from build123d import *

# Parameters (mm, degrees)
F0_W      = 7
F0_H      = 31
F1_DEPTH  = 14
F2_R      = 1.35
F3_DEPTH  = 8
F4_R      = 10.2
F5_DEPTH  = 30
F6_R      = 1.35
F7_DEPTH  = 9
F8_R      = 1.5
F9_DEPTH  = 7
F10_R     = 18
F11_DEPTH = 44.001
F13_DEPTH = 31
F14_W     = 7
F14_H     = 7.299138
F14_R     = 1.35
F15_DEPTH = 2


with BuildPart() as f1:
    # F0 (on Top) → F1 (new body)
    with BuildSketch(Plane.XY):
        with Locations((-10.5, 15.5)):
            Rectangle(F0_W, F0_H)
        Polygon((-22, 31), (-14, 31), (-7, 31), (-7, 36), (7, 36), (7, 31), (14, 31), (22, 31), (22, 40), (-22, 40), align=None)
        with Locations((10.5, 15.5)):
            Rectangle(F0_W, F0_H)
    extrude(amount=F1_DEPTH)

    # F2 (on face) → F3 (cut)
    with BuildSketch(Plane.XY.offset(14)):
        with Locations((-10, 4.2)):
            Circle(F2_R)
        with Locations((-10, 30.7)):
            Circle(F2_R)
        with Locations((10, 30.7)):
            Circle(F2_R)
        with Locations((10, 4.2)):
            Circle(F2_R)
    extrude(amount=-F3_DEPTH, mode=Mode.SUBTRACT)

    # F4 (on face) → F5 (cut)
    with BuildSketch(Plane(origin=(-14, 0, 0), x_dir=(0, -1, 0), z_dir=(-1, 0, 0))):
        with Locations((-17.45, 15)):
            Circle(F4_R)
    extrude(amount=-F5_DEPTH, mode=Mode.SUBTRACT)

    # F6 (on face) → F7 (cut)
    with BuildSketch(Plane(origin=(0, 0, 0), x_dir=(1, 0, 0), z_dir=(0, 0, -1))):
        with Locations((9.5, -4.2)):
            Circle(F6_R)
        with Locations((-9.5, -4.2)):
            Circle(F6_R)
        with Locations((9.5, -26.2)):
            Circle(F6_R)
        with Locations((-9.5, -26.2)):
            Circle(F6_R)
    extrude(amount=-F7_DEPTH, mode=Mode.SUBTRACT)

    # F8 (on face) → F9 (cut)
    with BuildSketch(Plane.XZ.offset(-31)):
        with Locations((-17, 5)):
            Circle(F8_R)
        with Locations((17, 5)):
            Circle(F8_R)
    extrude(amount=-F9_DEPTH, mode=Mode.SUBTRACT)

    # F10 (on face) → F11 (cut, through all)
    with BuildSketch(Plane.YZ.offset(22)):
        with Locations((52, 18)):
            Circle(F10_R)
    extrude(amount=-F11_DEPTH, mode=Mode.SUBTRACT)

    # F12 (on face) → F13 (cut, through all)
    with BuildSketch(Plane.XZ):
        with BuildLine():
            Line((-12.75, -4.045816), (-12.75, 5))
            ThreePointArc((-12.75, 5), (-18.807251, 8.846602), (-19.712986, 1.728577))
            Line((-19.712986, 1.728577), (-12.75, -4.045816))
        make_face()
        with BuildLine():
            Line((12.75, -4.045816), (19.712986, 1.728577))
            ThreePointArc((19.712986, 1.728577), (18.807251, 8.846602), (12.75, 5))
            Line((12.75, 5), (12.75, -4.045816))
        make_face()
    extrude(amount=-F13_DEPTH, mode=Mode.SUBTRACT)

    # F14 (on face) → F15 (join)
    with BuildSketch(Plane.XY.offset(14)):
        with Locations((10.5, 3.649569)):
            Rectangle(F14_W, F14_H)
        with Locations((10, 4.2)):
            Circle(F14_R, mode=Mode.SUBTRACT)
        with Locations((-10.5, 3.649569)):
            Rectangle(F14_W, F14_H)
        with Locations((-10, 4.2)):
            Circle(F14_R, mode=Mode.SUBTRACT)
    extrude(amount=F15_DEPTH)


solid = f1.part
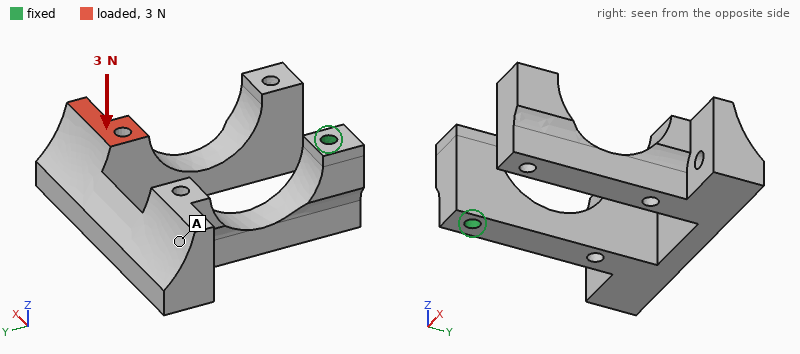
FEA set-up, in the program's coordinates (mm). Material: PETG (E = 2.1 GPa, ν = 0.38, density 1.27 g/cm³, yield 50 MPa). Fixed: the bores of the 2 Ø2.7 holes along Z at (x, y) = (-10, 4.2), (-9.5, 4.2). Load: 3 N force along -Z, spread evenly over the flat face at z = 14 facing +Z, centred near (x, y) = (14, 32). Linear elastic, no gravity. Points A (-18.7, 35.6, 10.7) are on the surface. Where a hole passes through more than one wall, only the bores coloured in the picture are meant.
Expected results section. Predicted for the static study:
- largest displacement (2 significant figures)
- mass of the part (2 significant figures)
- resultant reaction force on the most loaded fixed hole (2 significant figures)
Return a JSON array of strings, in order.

["0.63 mm", "8.2 g", "3.8 N"]
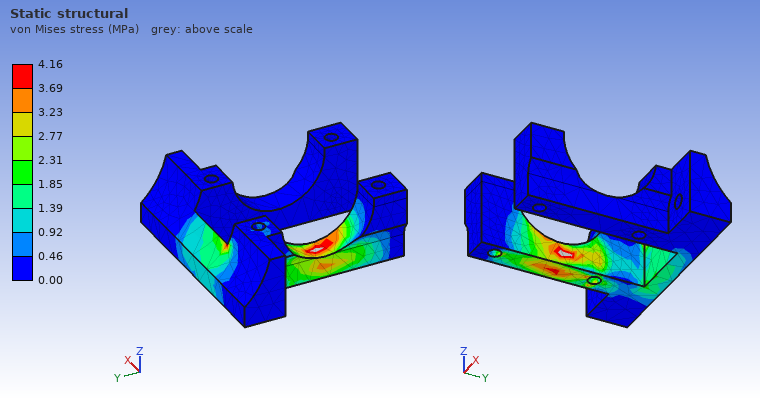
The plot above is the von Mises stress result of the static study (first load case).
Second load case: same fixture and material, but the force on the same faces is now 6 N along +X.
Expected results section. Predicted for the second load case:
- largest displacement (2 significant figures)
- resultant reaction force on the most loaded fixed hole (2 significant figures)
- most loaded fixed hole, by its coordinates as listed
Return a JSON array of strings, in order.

["0.65 mm", "7.0 N", "(-9.5, 4.2)"]
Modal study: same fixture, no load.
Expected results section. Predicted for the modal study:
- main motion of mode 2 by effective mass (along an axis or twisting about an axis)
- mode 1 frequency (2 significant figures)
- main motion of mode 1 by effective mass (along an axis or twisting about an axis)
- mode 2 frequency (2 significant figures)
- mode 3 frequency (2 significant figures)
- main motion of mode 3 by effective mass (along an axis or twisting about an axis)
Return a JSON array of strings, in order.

["along Z", "170 Hz", "along Y", "190 Hz", "290 Hz", "along X"]
